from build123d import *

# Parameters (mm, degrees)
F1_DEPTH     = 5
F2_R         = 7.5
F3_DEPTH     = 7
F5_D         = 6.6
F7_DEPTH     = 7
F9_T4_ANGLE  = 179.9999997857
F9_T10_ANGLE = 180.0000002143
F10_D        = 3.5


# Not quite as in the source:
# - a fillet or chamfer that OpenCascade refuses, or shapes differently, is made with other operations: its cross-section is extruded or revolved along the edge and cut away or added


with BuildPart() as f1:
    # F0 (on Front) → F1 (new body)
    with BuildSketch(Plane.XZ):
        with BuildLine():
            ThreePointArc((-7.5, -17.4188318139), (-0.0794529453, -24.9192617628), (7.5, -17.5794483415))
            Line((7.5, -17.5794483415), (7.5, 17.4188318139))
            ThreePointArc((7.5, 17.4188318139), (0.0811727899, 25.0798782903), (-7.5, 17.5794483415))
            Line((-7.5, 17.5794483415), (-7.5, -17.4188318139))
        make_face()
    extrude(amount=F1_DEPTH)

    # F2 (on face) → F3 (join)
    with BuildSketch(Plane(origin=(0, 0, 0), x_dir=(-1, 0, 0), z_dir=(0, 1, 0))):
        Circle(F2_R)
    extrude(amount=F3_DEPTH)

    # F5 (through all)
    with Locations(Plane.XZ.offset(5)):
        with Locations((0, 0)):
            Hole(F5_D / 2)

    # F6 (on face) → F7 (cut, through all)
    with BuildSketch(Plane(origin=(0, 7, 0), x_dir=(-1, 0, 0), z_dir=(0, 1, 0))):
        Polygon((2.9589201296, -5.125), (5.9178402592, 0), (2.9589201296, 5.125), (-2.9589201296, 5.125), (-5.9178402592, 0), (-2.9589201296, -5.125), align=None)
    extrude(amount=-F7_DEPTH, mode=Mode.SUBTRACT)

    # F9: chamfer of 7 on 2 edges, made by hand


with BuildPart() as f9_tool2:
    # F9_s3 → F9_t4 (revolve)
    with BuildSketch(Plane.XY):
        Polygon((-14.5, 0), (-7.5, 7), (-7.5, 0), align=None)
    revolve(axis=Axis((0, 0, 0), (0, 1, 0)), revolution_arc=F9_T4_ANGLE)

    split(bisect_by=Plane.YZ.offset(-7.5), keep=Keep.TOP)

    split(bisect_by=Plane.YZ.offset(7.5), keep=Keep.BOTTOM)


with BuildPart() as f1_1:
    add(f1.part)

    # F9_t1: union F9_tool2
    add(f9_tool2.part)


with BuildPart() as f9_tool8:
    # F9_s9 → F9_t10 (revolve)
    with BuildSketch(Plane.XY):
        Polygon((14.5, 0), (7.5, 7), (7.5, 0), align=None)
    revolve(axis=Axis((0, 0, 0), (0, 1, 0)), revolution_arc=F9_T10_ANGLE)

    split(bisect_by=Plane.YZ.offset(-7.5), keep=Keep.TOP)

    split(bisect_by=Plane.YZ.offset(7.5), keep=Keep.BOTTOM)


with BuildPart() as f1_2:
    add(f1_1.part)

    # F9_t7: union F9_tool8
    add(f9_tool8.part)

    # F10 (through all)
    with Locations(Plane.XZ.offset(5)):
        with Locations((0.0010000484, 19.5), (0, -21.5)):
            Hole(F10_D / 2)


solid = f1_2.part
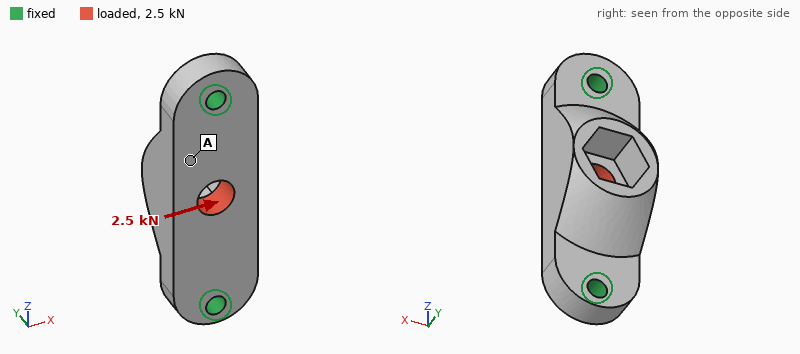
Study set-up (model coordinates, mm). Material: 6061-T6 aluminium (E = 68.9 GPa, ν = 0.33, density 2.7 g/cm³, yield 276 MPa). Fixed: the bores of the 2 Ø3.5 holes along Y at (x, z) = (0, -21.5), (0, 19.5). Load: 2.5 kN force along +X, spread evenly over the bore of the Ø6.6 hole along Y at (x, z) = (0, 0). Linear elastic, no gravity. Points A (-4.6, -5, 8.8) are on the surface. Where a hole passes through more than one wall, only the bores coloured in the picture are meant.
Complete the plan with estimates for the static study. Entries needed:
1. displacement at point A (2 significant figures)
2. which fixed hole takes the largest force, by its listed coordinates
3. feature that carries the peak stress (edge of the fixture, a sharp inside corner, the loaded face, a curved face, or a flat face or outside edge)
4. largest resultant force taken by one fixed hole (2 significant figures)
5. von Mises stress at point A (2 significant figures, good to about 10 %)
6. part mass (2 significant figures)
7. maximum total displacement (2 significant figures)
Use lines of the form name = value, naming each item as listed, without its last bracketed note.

displacement at point A = 17 µm
which fixed hole takes the largest force, by its listed coordinates = (0, 19.5)
feature that carries the peak stress = edge of the fixture
largest resultant force taken by one fixed hole = 1.3 kN
von Mises stress at point A = 28 MPa
part mass = 13 g
maximum total displacement = 28 µm
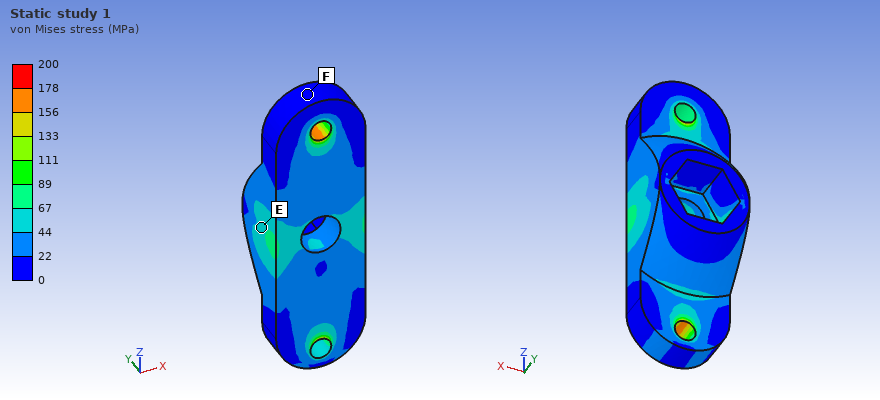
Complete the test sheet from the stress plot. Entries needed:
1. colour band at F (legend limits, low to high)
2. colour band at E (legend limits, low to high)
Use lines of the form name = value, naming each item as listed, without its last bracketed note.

colour band at F = 0 to 22 MPa
colour band at E = 44 to 67 MPa
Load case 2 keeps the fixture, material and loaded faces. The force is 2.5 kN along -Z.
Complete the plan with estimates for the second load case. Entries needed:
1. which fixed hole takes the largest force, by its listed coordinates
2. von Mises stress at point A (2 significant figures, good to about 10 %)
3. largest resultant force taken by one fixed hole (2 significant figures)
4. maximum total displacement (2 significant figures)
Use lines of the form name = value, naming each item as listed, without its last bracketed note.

which fixed hole takes the largest force, by its listed coordinates = (0, 19.5)
von Mises stress at point A = 21 MPa
largest resultant force taken by one fixed hole = 1.3 kN
maximum total displacement = 6.1 µm
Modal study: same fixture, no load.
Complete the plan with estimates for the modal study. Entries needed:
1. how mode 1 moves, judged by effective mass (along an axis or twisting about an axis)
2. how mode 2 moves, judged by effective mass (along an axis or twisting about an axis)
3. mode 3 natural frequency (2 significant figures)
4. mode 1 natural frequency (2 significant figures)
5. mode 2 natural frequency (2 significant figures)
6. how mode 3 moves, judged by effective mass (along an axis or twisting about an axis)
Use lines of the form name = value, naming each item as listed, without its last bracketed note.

how mode 1 moves, judged by effective mass = along X
how mode 2 moves, judged by effective mass = along Y
mode 3 natural frequency = 23 kHz
mode 1 natural frequency = 14 kHz
mode 2 natural frequency = 15 kHz
how mode 3 moves, judged by effective mass = along X
